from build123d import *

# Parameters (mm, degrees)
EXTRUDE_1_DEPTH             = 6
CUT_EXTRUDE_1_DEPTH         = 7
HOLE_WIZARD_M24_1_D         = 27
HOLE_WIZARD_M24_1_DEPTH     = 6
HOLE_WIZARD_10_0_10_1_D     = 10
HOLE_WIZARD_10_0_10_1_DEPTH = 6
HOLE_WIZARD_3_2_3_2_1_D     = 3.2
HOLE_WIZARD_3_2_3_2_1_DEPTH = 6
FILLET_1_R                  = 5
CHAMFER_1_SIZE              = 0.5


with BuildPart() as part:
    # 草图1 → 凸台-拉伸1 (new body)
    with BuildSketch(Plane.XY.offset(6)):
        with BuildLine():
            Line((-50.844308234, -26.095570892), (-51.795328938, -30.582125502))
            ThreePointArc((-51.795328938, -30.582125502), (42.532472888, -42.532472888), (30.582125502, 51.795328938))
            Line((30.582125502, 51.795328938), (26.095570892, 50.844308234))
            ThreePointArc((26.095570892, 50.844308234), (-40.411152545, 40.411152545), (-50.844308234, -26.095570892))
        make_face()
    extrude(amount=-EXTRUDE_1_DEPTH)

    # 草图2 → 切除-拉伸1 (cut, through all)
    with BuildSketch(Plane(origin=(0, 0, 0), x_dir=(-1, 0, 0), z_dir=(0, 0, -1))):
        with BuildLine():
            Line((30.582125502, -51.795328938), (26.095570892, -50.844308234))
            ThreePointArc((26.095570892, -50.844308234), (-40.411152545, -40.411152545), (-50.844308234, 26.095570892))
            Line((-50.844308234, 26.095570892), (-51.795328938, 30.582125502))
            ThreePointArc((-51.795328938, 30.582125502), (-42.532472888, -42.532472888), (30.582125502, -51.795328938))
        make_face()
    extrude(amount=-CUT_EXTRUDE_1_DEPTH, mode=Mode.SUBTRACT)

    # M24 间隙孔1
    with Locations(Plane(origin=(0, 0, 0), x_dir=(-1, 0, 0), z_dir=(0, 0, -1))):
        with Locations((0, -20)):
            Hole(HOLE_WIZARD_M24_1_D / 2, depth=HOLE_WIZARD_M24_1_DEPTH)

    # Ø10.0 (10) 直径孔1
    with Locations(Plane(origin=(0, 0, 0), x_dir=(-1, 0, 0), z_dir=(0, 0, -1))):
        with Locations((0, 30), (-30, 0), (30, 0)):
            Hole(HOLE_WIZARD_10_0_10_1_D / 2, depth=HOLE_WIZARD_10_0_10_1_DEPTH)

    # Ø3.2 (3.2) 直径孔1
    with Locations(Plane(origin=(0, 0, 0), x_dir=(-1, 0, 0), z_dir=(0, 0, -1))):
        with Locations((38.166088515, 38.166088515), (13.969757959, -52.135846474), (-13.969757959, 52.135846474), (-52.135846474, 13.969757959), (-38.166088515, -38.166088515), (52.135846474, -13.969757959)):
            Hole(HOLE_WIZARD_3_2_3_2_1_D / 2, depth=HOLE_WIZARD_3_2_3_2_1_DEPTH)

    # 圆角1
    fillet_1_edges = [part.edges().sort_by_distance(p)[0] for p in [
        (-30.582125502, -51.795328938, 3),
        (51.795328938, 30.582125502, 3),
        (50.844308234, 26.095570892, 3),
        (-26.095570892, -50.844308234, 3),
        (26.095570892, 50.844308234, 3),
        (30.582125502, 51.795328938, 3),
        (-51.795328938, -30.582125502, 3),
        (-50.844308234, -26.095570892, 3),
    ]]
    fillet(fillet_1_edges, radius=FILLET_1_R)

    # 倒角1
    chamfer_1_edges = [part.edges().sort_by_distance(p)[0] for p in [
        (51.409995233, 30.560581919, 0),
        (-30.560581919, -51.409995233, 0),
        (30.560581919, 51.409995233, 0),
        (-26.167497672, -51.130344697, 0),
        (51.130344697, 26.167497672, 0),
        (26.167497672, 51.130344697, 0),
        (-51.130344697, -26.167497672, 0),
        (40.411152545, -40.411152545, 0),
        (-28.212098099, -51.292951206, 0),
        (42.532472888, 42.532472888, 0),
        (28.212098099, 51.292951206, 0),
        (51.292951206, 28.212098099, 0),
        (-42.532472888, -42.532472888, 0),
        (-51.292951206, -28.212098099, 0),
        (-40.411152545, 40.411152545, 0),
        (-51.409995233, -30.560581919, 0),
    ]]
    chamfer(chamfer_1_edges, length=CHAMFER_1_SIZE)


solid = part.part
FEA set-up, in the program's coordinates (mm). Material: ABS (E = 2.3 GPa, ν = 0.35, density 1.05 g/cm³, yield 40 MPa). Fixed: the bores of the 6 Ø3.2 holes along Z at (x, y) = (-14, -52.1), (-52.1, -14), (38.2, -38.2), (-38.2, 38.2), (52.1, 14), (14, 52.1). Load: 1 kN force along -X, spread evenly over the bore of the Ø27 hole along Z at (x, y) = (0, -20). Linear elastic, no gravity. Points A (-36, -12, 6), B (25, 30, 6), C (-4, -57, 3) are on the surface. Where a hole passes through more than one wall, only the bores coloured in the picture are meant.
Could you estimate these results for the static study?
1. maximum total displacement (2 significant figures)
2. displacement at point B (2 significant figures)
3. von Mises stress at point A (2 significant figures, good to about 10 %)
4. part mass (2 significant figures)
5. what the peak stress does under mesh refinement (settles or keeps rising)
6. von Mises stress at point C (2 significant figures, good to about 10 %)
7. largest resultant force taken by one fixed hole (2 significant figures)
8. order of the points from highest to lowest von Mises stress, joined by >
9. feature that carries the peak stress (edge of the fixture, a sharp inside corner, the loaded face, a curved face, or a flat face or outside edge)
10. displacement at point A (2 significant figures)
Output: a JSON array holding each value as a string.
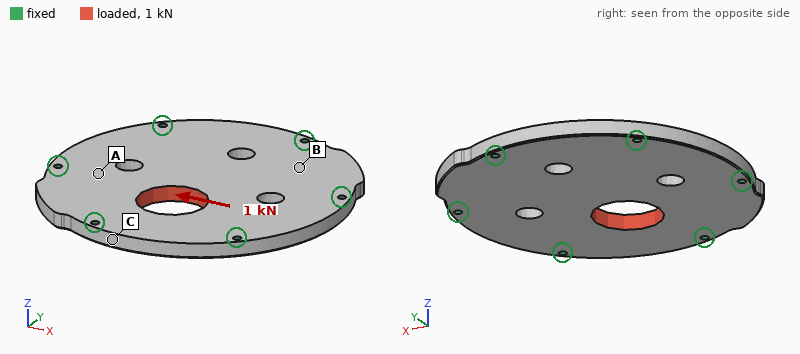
["43 µm", "12 µm", "2.2 MPa", "60 g", "keeps rising", "1.1 MPa", "260 N", "A > C > B", "edge of the fixture", "21 µm"]
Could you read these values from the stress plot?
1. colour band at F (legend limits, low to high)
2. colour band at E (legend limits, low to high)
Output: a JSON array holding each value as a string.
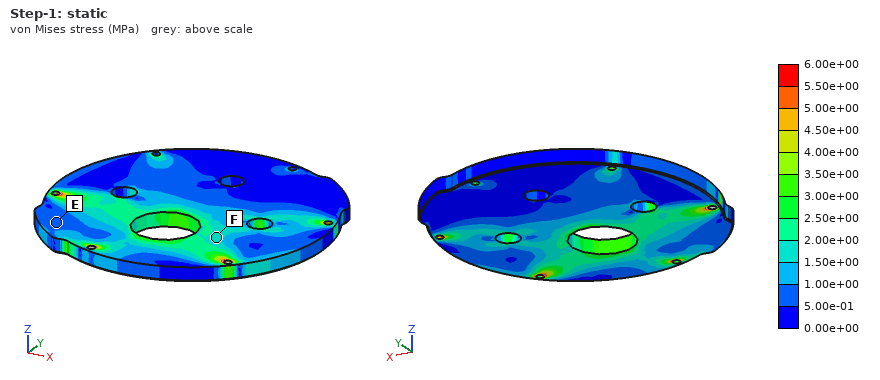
["1.50e+00 to 2.00e+00 MPa", "5.00e-01 to 1.00e+00 MPa"]
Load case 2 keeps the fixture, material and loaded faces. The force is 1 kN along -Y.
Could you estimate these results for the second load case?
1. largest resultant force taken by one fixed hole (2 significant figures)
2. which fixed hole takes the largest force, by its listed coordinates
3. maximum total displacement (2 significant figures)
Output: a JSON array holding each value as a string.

["320 N", "(-14, -52.1)", "51 µm"]
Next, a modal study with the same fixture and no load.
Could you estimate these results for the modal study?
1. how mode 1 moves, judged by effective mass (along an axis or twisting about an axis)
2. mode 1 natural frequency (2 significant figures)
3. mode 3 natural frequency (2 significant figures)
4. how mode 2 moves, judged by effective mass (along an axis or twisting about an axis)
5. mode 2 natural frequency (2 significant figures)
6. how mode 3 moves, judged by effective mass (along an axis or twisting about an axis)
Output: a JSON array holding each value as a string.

["along Z", "1100 Hz", "2200 Hz", "twisting about Y", "2100 Hz", "twisting about X"]
